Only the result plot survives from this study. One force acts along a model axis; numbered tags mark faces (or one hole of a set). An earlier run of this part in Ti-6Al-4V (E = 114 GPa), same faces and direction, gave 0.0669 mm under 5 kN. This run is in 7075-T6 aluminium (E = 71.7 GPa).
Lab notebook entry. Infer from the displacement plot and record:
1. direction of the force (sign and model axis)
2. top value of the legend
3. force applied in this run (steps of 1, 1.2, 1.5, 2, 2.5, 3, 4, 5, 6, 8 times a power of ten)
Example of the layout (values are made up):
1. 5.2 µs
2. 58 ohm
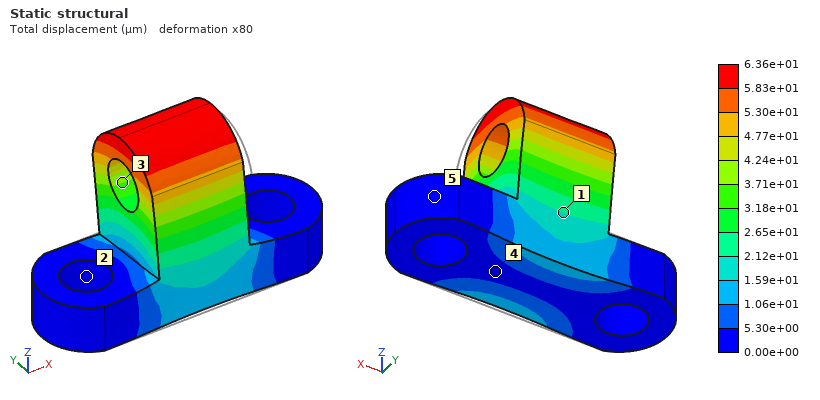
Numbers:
1. +Y
2. 6.36e+01 µm
3. 3 kN
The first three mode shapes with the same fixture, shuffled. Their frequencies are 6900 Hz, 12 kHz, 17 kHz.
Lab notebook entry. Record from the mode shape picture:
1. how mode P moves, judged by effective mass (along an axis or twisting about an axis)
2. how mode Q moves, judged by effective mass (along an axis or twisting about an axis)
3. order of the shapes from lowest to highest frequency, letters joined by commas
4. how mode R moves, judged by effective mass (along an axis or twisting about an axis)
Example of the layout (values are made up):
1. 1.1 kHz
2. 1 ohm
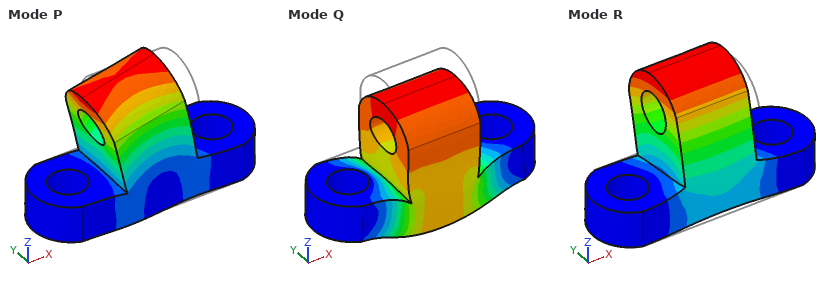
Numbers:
1. along X
2. along Z
3. R, P, Q
4. along Y
